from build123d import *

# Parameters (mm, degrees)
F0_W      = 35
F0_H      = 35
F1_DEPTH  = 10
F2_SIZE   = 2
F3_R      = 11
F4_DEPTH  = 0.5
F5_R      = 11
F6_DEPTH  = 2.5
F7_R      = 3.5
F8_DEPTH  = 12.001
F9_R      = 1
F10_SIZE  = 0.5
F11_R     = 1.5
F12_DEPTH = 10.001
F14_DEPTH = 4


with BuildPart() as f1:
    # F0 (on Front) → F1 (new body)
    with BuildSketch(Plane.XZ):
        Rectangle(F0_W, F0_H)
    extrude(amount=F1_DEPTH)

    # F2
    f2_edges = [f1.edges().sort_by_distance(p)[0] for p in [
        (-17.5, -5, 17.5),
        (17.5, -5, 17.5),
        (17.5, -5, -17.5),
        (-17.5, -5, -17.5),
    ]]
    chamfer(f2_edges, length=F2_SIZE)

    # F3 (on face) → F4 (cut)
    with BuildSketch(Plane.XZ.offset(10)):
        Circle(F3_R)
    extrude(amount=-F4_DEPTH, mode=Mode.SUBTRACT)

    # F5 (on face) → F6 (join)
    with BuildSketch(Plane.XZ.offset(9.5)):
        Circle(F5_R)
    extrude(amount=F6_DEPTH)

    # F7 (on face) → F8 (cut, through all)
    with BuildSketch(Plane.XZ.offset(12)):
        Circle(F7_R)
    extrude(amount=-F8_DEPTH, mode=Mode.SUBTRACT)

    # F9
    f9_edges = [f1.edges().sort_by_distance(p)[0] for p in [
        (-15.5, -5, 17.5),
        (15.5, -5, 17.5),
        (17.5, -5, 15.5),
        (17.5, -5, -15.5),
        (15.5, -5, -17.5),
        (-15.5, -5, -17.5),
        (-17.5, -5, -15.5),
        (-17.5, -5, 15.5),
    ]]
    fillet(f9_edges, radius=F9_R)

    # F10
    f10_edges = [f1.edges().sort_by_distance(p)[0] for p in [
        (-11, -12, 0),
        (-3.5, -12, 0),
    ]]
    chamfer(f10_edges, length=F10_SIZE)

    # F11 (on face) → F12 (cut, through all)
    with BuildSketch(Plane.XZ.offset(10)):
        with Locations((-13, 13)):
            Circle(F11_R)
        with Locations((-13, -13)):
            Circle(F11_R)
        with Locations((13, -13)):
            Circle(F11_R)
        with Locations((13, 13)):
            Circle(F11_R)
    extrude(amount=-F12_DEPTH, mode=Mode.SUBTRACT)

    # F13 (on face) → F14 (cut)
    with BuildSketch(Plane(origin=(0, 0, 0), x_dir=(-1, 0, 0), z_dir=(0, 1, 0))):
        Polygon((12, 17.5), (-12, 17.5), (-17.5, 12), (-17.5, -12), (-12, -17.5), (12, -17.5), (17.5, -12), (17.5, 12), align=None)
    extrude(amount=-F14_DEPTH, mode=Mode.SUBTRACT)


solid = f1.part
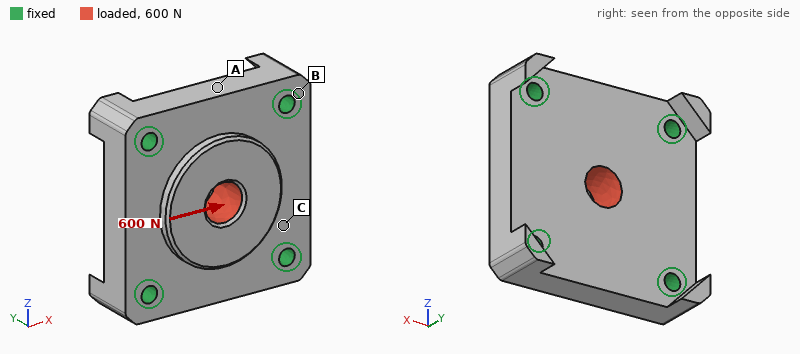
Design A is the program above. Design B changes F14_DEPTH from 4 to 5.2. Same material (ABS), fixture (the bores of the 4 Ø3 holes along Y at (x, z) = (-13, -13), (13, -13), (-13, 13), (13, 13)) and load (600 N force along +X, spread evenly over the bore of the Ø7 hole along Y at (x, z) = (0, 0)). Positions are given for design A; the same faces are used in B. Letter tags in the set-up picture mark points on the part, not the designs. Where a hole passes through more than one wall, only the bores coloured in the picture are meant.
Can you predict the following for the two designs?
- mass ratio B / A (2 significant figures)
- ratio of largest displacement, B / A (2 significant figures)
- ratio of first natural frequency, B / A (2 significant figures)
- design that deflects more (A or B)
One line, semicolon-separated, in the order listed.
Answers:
0.83; 1.2; 0.88; B
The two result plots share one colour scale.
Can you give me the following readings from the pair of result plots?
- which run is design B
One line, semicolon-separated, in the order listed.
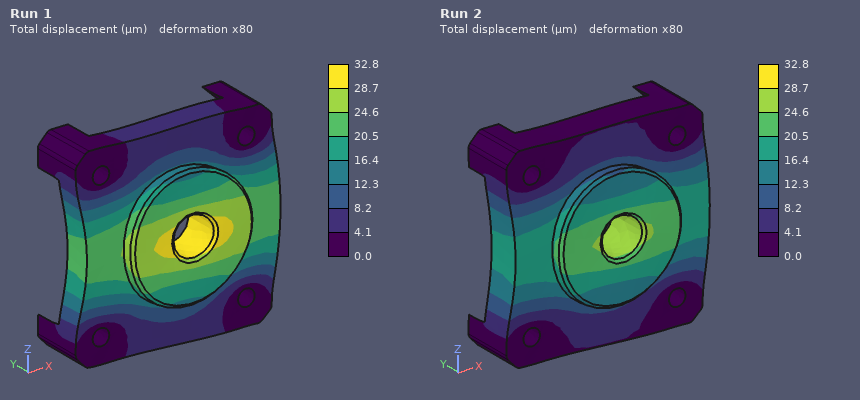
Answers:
Run 1
